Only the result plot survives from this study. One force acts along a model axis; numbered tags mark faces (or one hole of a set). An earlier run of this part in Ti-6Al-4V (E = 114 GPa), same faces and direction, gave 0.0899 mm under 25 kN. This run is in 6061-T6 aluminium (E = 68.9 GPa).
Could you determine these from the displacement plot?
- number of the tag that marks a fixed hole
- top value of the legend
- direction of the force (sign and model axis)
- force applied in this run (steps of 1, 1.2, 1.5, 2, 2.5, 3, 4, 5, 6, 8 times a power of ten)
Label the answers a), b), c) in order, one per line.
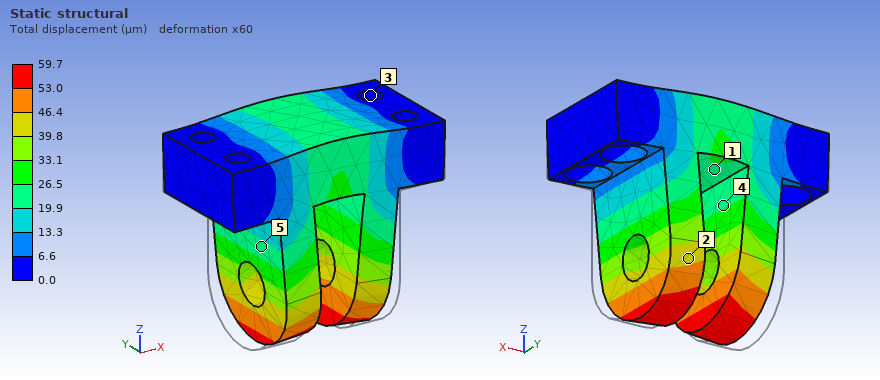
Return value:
a) 3
b) 59.7 µm
c) +Z
d) 10 kN
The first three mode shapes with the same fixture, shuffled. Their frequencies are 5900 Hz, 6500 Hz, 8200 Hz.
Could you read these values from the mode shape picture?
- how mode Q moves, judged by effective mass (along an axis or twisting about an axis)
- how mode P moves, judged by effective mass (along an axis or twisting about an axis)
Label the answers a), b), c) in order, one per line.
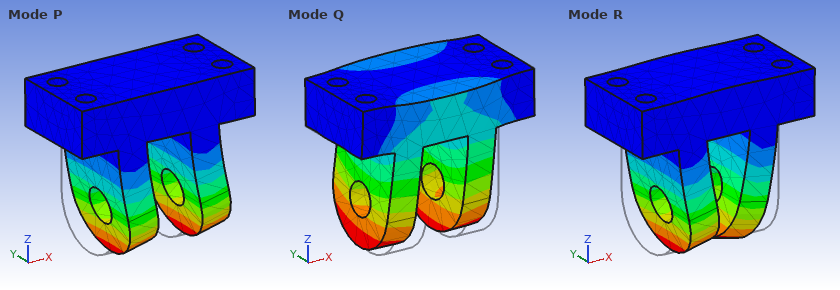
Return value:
a) along Y
b) along X
